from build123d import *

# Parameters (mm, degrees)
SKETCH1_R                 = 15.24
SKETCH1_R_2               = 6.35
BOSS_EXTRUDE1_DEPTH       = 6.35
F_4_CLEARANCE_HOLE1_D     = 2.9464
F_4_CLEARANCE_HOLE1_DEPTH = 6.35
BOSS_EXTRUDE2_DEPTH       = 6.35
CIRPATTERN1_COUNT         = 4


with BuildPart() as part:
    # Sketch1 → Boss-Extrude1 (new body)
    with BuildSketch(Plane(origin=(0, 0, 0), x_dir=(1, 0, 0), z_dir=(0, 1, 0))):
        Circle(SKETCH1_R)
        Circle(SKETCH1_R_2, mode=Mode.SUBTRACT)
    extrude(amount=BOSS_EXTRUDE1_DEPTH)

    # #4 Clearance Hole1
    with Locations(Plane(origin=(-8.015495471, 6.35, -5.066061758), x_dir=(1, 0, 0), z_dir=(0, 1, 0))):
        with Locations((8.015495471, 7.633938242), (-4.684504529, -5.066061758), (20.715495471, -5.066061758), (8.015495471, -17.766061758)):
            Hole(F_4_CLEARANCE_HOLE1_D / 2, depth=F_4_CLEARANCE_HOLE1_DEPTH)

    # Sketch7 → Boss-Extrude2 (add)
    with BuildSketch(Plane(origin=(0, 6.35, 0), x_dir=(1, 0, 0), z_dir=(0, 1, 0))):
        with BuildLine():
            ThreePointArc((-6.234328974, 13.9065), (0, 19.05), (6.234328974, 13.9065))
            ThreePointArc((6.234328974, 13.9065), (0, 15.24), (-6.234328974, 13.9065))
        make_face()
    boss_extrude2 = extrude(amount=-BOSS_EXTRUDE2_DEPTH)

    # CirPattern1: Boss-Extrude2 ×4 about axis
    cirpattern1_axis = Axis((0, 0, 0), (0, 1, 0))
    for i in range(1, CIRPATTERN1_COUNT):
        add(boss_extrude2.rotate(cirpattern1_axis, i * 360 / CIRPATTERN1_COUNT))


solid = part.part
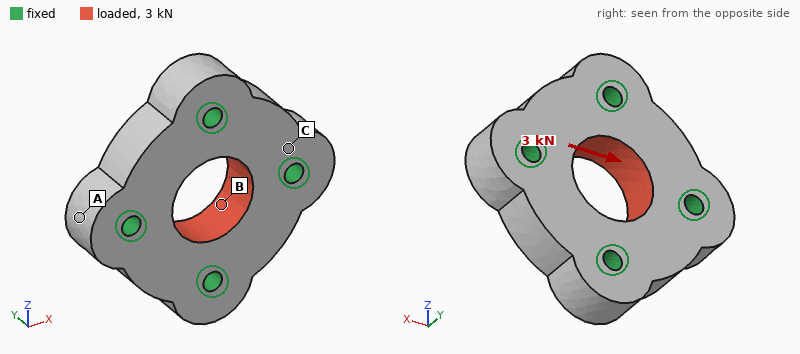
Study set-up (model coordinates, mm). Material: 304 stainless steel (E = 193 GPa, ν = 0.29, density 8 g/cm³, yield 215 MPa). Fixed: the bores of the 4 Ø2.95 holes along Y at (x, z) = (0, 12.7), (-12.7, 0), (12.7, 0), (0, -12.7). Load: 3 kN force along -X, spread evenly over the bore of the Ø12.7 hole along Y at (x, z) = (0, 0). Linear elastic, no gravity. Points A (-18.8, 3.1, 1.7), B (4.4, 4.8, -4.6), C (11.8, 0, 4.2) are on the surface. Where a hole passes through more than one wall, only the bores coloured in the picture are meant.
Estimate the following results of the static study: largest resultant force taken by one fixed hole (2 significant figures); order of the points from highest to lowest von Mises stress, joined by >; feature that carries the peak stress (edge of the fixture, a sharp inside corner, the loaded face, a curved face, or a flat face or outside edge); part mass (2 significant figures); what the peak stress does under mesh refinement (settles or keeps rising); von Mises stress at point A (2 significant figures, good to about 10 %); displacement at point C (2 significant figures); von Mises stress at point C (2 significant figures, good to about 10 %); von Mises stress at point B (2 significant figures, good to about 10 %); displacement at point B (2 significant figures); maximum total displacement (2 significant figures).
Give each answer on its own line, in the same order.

900 N
B > C > A
edge of the fixture
37 g
keeps rising
4.5 MPa
0.33 µm
9.5 MPa
16 MPa
0.78 µm
0.84 µm
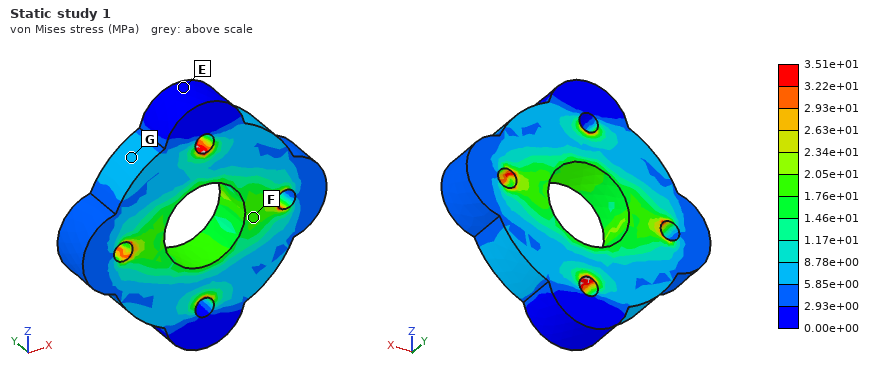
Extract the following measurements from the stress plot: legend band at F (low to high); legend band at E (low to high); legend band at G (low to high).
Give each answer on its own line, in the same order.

1.76e+01 to 2.05e+01 MPa
0.00e+00 to 2.93e+00 MPa
5.85e+00 to 8.78e+00 MPa
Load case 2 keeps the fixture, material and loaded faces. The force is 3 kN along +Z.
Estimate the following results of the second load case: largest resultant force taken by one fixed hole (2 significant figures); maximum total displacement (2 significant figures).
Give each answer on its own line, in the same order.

900 N
0.84 µm
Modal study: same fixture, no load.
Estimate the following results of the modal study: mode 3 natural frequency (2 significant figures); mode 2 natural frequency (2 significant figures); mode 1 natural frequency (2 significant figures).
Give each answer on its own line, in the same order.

59 kHz
59 kHz
56 kHz
